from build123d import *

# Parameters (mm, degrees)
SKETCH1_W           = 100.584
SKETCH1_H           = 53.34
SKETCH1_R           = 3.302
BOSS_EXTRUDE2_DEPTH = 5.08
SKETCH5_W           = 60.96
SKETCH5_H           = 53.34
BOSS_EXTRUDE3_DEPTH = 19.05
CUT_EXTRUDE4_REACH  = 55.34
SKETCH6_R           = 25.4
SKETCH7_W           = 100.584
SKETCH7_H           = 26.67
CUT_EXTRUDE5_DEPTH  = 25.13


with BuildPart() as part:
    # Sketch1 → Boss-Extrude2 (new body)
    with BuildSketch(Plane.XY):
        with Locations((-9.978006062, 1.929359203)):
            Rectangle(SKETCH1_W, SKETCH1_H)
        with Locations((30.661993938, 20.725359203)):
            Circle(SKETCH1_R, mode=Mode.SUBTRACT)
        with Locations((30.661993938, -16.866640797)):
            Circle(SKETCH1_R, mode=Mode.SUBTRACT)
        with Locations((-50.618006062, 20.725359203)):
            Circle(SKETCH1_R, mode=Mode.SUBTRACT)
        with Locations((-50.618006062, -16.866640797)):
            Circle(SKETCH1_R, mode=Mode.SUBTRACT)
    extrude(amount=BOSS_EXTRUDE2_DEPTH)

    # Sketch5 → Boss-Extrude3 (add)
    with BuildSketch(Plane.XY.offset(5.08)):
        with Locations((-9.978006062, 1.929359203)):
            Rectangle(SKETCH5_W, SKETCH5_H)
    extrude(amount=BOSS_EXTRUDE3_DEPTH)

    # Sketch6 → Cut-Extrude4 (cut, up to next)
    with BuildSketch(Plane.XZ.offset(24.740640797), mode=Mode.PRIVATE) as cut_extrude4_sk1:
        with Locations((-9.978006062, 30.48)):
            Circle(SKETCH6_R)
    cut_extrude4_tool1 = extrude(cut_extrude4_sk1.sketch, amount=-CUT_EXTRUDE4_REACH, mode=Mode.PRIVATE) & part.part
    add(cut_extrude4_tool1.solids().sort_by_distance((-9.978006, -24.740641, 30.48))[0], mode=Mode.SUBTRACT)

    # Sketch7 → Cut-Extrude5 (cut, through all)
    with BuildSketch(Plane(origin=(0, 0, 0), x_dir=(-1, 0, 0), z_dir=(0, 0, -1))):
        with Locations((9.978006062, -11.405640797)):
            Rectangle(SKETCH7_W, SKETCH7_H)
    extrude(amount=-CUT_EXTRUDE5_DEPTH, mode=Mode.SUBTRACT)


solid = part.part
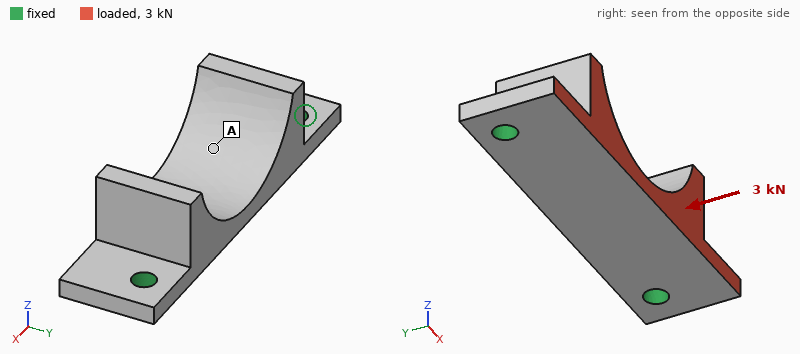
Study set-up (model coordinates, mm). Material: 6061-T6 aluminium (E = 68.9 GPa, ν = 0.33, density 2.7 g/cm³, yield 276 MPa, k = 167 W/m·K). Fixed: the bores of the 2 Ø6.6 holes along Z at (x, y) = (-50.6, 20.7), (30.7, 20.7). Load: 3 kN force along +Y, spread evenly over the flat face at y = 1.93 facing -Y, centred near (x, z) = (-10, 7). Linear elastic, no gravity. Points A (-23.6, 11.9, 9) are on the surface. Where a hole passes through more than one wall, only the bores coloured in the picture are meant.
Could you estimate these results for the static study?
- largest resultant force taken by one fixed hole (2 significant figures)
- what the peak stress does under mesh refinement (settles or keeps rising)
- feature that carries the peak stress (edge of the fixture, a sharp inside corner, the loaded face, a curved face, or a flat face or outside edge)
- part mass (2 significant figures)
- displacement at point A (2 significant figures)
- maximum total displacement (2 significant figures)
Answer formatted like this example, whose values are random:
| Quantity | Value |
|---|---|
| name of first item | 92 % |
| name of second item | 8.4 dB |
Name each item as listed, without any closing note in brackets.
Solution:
| Quantity | Value |
|---|---|
| largest resultant force taken by one fixed hole | 1.6 kN |
| what the peak stress does under mesh refinement | keeps rising |
| feature that carries the peak stress | edge of the fixture |
| part mass | 69 g |
| displacement at point A | 36 µm |
| maximum total displacement | 72 µm |
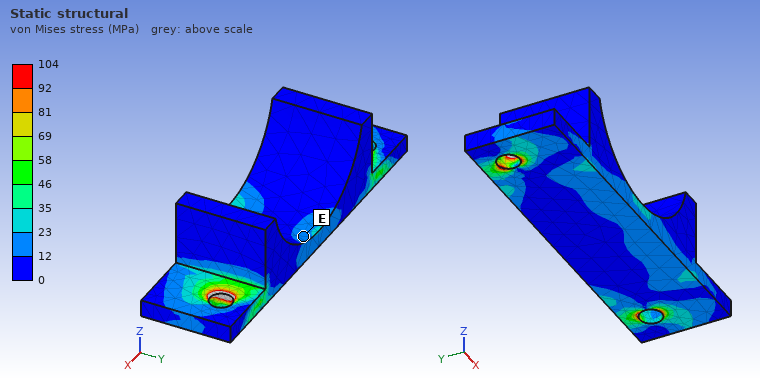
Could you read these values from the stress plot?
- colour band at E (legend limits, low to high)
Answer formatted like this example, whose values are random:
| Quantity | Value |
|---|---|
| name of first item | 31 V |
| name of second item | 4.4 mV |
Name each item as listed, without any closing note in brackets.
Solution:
| Quantity | Value |
|---|---|
| colour band at E | 12 to 23 MPa |
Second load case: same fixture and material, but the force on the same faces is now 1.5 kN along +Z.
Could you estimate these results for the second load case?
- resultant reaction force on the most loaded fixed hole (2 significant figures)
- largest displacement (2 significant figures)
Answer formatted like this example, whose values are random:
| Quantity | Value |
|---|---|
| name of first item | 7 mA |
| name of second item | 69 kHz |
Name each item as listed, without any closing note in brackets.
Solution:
| Quantity | Value |
|---|---|
| resultant reaction force on the most loaded fixed hole | 800 N |
| largest displacement | 0.15 mm |
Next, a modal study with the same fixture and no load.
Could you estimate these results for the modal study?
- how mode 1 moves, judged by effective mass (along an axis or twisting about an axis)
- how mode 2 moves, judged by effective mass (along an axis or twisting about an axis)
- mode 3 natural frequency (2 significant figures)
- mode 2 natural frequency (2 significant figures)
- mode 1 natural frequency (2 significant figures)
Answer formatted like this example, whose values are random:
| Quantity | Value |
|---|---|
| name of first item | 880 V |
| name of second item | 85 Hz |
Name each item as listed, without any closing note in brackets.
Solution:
| Quantity | Value |
|---|---|
| how mode 1 moves, judged by effective mass | along Z |
| how mode 2 moves, judged by effective mass | along Y |
| mode 3 natural frequency | 6600 Hz |
| mode 2 natural frequency | 4600 Hz |
| mode 1 natural frequency | 3000 Hz |
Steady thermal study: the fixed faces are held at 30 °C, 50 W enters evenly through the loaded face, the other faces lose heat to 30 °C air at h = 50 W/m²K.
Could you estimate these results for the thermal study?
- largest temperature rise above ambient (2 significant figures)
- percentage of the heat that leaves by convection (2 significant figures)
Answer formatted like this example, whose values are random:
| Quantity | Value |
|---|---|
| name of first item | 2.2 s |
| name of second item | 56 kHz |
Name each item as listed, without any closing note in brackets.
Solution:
| Quantity | Value |
|---|---|
| largest temperature rise above ambient | 19 K |
| percentage of the heat that leaves by convection | 9.5 % |
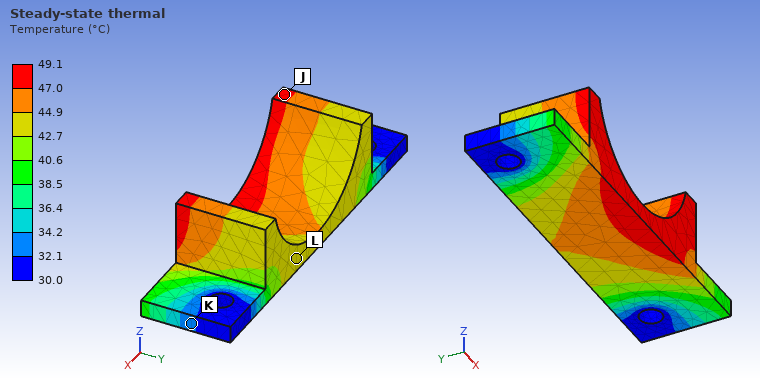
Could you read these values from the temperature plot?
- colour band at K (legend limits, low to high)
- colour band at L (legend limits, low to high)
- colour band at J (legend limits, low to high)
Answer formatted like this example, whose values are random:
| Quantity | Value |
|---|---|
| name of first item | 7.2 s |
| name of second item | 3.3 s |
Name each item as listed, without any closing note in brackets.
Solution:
| Quantity | Value |
|---|---|
| colour band at K | 32.1 to 34.2 °C |
| colour band at L | 42.7 to 44.9 °C |
| colour band at J | 47.0 to 49.1 °C |
